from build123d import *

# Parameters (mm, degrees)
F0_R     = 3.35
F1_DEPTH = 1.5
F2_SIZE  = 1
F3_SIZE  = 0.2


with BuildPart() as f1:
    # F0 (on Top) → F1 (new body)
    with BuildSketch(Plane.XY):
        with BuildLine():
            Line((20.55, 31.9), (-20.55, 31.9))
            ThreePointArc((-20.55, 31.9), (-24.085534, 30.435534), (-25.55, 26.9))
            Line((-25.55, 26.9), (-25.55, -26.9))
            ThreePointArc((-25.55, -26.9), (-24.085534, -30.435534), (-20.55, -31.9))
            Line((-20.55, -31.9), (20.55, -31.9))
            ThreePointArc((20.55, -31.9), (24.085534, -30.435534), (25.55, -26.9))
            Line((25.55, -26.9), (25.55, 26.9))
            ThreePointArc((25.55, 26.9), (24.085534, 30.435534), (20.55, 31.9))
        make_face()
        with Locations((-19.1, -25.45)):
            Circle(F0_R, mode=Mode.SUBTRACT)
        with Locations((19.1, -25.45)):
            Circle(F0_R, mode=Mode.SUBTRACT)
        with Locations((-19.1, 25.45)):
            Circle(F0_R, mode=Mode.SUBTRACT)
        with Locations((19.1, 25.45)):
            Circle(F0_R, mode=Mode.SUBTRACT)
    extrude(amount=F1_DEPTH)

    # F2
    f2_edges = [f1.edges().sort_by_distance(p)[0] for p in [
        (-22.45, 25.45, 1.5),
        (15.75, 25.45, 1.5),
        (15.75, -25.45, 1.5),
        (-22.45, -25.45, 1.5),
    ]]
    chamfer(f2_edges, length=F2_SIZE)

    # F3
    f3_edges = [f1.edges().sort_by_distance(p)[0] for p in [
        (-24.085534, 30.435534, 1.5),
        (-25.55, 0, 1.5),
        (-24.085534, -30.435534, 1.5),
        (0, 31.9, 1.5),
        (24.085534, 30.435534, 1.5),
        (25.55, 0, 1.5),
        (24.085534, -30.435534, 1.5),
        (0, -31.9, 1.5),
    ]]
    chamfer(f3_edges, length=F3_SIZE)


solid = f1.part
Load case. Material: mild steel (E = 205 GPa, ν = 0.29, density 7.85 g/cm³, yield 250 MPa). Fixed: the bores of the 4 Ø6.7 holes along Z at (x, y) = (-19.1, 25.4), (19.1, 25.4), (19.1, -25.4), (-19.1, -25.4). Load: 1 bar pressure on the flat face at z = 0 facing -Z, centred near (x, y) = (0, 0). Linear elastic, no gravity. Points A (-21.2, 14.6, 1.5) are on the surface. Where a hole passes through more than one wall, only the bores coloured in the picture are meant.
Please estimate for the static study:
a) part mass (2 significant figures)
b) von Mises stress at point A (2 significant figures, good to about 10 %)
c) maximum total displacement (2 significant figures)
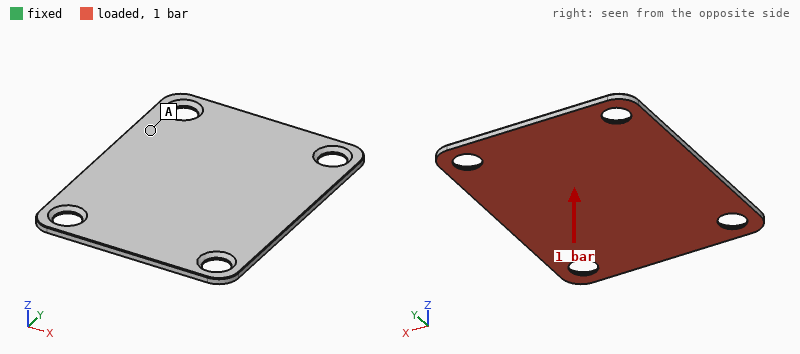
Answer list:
36 g
12 MPa
42 µm
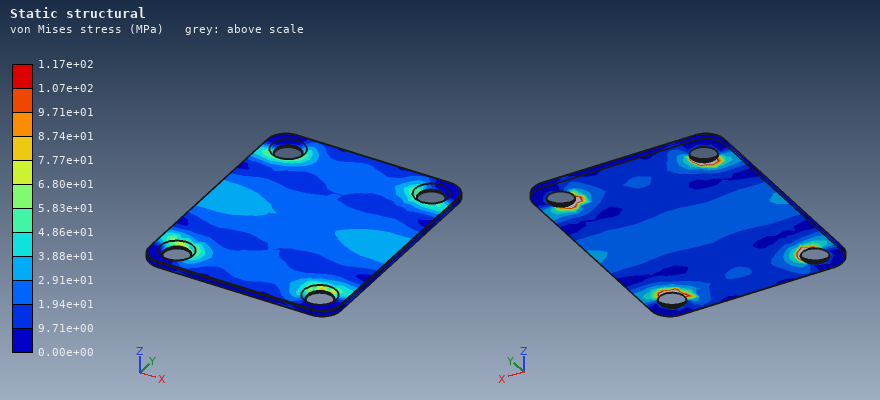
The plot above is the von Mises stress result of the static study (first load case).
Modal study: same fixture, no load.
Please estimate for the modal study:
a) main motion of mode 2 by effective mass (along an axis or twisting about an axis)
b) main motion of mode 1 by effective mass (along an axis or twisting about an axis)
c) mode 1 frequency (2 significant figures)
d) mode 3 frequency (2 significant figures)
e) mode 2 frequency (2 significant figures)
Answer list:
twisting about Y
along Z
2700 Hz
5200 Hz
3800 Hz
